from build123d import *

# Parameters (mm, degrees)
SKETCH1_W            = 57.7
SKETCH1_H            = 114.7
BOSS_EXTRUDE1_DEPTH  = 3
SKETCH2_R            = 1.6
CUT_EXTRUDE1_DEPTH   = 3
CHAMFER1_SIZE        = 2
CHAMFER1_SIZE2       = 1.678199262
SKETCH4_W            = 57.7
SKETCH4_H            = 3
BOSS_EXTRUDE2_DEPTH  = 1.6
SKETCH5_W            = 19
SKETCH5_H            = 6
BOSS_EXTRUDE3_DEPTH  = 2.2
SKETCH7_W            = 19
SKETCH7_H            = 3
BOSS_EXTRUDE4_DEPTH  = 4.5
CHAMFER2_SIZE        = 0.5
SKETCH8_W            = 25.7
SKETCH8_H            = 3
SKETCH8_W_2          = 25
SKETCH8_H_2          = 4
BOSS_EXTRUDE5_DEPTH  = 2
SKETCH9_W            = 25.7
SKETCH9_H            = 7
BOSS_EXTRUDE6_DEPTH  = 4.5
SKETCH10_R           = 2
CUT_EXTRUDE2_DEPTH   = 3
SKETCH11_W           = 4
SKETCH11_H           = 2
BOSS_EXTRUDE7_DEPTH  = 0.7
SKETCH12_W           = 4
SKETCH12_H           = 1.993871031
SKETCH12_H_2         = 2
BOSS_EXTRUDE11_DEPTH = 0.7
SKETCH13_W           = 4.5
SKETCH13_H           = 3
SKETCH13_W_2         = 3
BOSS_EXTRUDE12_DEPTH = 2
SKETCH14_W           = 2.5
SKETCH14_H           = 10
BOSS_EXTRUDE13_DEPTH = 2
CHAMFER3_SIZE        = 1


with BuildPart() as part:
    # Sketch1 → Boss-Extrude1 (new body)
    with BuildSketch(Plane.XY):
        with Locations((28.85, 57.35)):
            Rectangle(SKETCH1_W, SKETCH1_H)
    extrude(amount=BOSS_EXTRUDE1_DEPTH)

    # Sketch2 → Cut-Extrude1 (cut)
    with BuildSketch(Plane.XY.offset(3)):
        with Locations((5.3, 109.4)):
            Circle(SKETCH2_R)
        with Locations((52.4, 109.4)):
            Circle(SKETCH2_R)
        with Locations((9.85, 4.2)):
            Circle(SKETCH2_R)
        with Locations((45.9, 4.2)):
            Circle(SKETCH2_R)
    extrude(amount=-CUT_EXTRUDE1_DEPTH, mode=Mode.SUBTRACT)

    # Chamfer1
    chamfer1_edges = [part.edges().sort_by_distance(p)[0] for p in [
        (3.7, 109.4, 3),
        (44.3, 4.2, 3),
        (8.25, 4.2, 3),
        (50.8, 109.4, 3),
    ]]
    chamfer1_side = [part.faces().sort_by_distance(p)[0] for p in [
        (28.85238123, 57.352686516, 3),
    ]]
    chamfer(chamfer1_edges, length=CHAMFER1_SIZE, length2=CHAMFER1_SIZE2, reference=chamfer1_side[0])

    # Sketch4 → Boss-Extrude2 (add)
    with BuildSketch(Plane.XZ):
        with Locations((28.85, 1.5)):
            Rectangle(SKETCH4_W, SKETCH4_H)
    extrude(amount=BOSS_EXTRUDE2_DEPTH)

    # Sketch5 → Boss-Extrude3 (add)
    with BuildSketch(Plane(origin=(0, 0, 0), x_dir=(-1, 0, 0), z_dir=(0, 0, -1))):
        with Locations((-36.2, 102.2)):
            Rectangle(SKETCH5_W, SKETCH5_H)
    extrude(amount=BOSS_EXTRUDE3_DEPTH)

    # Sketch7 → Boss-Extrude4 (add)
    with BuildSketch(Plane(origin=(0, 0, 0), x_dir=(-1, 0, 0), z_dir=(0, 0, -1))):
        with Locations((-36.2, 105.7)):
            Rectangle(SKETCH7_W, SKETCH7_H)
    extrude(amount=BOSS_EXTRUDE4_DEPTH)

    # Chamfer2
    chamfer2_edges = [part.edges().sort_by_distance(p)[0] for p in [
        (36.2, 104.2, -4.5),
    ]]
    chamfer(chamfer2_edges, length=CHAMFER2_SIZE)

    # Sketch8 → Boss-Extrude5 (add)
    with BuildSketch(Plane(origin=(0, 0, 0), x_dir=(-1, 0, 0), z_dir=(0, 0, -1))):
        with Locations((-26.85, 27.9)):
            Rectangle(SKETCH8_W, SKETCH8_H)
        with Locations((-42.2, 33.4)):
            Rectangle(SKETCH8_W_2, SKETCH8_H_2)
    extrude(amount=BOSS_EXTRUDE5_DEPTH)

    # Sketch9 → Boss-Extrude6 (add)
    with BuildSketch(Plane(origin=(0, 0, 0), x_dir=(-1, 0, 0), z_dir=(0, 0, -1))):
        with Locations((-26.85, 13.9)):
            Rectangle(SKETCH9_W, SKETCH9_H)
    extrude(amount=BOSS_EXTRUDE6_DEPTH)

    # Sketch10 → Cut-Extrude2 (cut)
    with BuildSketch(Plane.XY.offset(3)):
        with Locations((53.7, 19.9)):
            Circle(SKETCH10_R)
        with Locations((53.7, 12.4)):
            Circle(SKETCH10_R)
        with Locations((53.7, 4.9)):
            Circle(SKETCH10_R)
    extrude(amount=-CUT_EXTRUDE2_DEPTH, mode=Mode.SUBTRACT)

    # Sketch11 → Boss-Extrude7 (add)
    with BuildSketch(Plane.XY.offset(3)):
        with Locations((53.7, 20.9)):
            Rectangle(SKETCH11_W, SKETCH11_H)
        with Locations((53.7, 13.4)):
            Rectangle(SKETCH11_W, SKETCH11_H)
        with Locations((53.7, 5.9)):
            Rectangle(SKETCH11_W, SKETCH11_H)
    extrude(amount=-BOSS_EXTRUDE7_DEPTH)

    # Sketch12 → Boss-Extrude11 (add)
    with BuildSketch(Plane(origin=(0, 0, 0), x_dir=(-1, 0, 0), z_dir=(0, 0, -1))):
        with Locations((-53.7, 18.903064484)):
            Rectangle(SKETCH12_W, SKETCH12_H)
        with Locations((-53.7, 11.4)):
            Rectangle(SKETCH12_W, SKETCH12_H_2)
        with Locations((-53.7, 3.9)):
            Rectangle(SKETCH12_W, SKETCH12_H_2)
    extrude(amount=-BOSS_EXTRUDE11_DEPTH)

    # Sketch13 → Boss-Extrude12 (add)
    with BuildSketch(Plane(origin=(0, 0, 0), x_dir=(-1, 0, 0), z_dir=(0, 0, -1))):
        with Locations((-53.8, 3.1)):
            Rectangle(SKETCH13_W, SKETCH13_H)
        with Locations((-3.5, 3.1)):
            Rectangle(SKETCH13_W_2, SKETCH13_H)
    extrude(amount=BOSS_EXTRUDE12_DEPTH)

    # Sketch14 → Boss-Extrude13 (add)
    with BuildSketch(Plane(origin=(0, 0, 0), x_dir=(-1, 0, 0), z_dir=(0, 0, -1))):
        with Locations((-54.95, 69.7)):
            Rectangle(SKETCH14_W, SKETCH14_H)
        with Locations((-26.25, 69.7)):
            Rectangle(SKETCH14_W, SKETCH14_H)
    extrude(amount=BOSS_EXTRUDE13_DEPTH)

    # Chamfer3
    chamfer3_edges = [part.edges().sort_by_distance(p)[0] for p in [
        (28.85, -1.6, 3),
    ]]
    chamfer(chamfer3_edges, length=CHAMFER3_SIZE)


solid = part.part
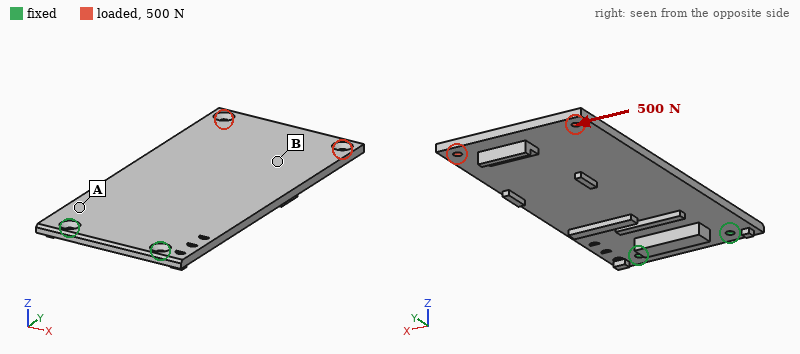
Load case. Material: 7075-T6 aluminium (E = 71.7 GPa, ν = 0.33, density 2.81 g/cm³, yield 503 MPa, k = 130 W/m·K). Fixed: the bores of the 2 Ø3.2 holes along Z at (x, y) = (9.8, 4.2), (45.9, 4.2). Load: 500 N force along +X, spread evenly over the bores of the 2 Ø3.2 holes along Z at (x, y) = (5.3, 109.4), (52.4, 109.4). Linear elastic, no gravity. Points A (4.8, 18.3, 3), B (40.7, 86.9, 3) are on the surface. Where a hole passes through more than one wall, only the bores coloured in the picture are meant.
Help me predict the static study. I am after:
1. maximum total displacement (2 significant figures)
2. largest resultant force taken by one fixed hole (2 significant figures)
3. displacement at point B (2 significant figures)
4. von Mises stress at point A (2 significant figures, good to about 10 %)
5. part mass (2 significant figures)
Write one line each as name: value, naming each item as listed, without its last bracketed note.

maximum total displacement: 0.15 mm
largest resultant force taken by one fixed hole: 1.4 kN
displacement at point B: 0.080 mm
von Mises stress at point A: 23 MPa
part mass: 61 g
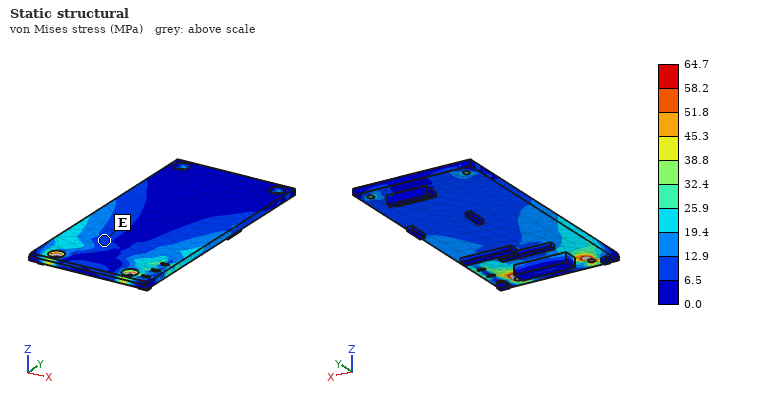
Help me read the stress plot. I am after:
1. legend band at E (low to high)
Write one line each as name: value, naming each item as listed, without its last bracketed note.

legend band at E: 6.5 to 12.9 MPa
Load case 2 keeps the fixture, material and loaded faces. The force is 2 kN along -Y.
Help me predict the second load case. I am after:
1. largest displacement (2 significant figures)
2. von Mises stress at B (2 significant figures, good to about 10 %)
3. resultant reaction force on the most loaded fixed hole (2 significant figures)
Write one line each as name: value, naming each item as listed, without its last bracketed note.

largest displacement: 1.0 mm
von Mises stress at B: 11 MPa
resultant reaction force on the most loaded fixed hole: 1.1 kN
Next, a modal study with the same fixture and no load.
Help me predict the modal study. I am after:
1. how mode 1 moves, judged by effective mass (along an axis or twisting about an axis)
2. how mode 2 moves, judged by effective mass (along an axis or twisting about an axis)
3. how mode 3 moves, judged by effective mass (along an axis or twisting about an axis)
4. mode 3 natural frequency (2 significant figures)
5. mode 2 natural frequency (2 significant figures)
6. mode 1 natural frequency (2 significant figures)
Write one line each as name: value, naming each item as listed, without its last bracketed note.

how mode 1 moves, judged by effective mass: along Z
how mode 2 moves, judged by effective mass: twisting about Y
how mode 3 moves, judged by effective mass: along Z
mode 3 natural frequency: 1100 Hz
mode 2 natural frequency: 850 Hz
mode 1 natural frequency: 170 Hz
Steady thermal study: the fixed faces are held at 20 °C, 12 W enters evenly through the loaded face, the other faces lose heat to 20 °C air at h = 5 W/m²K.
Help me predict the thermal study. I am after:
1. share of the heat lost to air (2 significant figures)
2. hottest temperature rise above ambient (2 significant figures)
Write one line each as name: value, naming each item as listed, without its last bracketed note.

share of the heat lost to air: 17 %
hottest temperature rise above ambient: 62 K
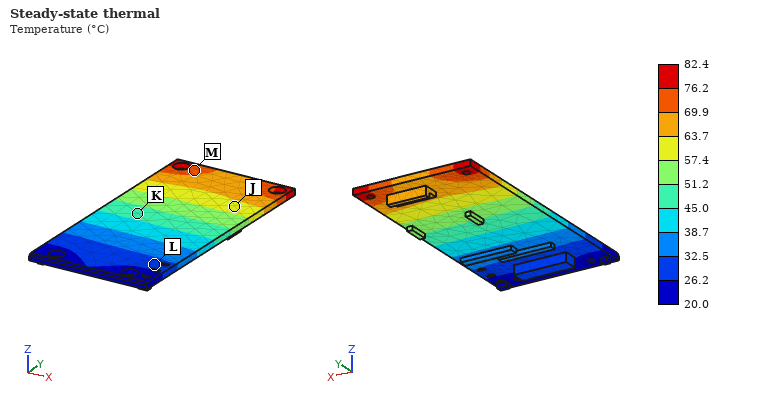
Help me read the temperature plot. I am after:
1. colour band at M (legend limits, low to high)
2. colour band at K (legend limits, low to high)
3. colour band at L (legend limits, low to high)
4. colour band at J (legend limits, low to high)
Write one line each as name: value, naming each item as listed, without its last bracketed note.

colour band at M: 69.9 to 76.2 °C
colour band at K: 45.0 to 51.2 °C
colour band at L: 26.2 to 32.5 °C
colour band at J: 57.4 to 63.7 °C
